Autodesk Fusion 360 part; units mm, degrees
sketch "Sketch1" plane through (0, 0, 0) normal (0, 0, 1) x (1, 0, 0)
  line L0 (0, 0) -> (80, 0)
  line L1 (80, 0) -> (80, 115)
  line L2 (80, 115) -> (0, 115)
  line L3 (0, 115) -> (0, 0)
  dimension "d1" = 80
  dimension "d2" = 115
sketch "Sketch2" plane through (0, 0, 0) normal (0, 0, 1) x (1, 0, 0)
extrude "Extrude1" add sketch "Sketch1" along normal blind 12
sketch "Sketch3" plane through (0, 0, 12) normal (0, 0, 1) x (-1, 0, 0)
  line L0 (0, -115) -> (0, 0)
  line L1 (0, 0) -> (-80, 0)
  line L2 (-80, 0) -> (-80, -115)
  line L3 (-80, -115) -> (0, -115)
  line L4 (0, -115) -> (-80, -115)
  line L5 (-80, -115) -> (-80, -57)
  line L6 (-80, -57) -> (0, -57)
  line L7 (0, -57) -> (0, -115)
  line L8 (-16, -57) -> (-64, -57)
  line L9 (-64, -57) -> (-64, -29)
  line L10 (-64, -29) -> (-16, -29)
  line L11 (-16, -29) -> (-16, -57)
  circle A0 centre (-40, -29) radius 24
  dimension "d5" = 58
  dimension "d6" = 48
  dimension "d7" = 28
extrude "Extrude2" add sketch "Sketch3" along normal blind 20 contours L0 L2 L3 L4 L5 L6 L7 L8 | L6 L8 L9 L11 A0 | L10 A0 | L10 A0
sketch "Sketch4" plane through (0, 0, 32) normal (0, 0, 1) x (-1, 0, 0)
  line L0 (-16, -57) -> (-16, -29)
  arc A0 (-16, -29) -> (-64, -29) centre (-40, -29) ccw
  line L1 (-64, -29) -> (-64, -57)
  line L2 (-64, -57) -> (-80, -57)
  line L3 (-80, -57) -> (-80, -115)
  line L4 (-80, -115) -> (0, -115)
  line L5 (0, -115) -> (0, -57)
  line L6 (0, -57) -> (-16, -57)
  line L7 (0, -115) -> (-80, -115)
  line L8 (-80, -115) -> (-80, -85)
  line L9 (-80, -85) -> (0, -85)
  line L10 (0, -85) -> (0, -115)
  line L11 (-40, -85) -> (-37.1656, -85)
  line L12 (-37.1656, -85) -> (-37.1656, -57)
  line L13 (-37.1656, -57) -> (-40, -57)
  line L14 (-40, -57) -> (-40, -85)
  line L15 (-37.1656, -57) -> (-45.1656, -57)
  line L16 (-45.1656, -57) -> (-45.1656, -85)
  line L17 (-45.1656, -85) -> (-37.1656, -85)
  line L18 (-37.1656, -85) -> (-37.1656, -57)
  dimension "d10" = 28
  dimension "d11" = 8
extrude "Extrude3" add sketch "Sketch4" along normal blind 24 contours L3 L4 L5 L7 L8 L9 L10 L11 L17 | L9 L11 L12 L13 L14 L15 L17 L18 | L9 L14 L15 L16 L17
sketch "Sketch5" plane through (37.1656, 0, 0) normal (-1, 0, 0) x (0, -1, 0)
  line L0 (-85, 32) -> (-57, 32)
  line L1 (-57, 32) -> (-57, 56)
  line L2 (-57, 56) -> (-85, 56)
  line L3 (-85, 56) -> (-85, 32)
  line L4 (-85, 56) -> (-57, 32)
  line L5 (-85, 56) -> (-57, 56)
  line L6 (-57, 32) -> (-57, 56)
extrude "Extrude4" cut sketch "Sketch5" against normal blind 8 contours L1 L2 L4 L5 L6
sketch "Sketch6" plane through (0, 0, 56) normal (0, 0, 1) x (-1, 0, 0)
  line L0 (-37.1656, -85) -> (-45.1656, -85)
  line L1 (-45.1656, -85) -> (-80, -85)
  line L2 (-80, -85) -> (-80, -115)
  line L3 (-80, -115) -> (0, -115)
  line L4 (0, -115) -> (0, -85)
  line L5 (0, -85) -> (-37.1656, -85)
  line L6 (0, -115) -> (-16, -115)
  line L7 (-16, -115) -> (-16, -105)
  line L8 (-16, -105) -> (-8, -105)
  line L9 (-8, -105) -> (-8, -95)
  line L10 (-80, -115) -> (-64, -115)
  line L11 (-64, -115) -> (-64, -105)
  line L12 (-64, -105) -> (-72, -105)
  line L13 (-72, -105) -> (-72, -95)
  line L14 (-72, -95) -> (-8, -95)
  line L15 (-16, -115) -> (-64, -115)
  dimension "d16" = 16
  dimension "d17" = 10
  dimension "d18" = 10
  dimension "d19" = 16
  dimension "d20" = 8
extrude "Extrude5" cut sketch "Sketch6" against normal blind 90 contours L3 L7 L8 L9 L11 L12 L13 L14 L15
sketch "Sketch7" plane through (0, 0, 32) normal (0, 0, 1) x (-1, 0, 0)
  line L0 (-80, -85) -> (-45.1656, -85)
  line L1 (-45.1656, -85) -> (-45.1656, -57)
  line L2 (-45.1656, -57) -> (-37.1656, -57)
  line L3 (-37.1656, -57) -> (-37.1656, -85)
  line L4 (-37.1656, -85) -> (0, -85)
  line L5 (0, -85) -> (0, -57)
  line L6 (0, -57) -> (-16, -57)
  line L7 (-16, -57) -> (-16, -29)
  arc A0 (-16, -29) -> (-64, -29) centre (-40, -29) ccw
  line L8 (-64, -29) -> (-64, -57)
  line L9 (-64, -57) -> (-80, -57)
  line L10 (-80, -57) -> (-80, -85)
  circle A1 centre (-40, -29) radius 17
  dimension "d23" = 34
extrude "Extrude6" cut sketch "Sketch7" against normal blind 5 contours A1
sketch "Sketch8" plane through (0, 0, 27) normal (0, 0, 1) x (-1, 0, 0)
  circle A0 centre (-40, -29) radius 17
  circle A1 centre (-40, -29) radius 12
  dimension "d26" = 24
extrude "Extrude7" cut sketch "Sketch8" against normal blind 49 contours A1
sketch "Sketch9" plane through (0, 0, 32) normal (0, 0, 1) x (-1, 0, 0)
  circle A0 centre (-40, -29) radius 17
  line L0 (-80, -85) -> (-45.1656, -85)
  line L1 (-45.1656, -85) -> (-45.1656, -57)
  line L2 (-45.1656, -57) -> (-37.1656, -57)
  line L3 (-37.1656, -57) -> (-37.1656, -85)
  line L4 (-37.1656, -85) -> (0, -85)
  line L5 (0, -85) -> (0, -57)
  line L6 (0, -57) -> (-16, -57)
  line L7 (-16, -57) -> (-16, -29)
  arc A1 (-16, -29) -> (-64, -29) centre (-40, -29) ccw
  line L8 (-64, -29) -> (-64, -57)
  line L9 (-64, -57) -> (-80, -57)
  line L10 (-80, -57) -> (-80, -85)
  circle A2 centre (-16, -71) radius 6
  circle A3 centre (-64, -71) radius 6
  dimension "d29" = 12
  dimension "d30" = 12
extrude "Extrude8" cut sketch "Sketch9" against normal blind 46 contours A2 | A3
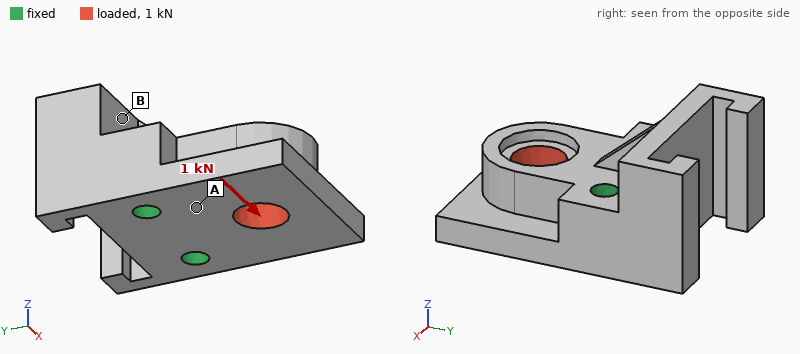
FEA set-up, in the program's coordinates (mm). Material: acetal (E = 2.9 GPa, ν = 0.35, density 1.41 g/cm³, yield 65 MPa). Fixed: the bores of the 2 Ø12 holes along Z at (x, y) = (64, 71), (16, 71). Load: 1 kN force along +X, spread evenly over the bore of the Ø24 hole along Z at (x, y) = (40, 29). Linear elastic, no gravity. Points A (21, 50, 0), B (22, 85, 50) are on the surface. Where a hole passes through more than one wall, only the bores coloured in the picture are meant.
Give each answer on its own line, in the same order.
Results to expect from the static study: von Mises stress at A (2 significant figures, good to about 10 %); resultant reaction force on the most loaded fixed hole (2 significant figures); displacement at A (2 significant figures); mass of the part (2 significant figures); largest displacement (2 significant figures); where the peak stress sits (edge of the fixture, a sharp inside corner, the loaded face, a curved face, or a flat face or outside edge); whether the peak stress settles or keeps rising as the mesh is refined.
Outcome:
0.89 MPa
900 N
12 µm
310 g
66 µm
edge of the fixture
keeps rising
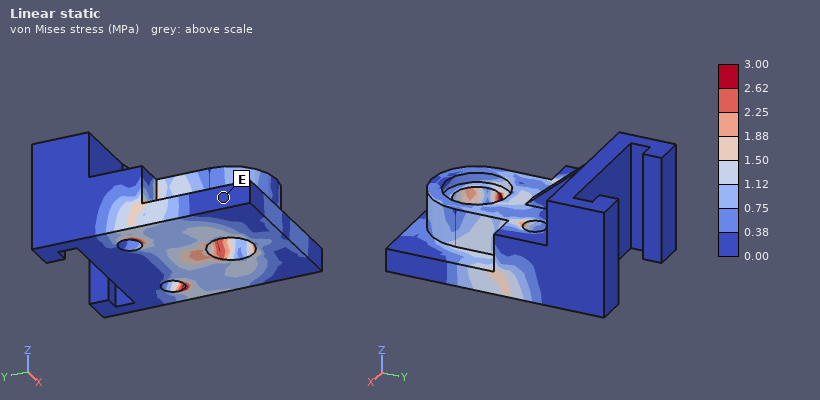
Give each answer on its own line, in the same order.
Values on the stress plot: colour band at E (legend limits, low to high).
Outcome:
0.00 to 0.38 MPa
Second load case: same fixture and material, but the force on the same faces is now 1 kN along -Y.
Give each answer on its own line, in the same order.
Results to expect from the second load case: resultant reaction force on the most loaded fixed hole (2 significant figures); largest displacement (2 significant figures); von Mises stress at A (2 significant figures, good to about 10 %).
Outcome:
510 N
18 µm
0.75 MPa
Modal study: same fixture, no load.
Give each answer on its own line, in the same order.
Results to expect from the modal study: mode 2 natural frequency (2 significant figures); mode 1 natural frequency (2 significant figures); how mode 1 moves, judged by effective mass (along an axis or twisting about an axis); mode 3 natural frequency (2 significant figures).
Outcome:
1800 Hz
1400 Hz
along Z
1800 Hz
